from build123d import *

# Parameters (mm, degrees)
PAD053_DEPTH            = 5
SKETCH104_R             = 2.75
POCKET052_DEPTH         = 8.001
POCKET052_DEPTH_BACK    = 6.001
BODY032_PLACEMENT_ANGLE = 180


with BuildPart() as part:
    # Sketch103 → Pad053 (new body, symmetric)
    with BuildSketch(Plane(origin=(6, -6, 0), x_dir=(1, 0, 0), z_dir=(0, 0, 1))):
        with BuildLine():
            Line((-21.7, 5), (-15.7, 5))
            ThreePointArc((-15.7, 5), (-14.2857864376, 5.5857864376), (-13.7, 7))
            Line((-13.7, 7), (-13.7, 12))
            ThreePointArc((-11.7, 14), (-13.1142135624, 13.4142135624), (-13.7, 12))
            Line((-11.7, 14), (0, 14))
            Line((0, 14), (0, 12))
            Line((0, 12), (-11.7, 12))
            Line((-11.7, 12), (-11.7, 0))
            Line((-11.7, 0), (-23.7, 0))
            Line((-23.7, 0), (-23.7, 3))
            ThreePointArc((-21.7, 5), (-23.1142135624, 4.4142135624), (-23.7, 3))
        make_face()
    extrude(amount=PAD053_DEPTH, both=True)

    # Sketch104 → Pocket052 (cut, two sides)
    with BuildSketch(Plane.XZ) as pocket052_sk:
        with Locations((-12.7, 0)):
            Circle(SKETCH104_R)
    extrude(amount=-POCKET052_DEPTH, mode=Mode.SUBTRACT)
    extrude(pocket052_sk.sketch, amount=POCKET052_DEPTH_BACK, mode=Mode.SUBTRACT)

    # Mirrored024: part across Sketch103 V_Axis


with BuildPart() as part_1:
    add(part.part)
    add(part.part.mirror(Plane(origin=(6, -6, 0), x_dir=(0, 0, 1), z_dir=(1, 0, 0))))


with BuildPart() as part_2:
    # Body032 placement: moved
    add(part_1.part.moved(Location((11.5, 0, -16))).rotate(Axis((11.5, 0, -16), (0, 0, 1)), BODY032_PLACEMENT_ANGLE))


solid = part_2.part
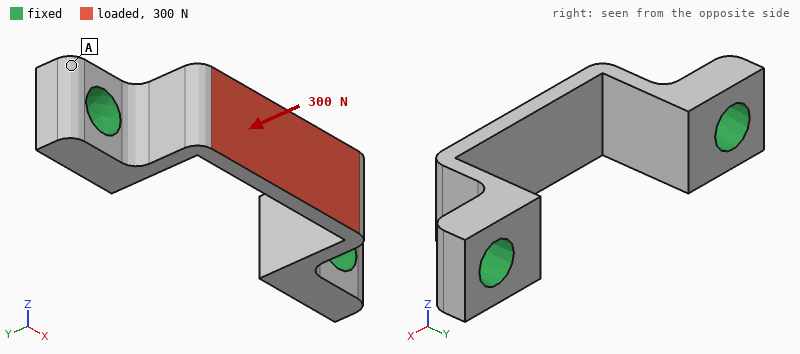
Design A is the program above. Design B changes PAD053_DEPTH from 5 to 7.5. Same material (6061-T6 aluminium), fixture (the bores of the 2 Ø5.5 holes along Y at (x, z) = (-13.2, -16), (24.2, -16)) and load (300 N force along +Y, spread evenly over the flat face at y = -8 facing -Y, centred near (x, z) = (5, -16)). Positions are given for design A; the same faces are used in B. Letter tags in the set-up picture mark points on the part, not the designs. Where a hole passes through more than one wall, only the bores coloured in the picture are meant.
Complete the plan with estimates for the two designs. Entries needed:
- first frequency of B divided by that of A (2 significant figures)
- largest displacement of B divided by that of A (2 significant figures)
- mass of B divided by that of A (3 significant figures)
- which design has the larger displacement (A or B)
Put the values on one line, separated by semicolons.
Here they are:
1.00; 0.68; 1.57; A
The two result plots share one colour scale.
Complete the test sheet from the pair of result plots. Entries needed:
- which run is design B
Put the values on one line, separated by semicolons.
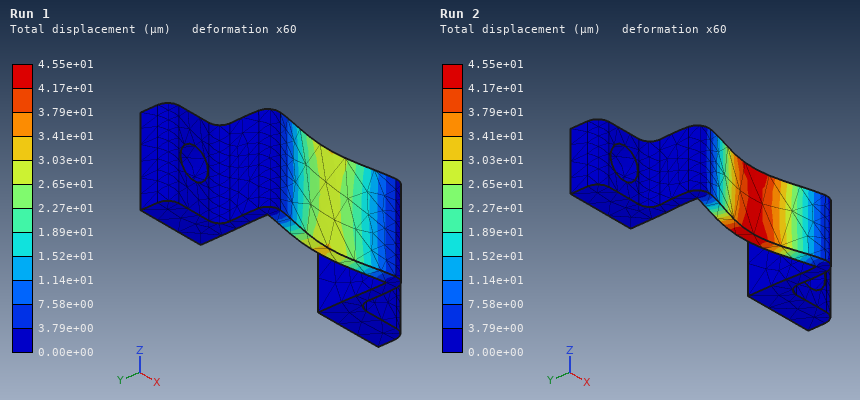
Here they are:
Run 1
